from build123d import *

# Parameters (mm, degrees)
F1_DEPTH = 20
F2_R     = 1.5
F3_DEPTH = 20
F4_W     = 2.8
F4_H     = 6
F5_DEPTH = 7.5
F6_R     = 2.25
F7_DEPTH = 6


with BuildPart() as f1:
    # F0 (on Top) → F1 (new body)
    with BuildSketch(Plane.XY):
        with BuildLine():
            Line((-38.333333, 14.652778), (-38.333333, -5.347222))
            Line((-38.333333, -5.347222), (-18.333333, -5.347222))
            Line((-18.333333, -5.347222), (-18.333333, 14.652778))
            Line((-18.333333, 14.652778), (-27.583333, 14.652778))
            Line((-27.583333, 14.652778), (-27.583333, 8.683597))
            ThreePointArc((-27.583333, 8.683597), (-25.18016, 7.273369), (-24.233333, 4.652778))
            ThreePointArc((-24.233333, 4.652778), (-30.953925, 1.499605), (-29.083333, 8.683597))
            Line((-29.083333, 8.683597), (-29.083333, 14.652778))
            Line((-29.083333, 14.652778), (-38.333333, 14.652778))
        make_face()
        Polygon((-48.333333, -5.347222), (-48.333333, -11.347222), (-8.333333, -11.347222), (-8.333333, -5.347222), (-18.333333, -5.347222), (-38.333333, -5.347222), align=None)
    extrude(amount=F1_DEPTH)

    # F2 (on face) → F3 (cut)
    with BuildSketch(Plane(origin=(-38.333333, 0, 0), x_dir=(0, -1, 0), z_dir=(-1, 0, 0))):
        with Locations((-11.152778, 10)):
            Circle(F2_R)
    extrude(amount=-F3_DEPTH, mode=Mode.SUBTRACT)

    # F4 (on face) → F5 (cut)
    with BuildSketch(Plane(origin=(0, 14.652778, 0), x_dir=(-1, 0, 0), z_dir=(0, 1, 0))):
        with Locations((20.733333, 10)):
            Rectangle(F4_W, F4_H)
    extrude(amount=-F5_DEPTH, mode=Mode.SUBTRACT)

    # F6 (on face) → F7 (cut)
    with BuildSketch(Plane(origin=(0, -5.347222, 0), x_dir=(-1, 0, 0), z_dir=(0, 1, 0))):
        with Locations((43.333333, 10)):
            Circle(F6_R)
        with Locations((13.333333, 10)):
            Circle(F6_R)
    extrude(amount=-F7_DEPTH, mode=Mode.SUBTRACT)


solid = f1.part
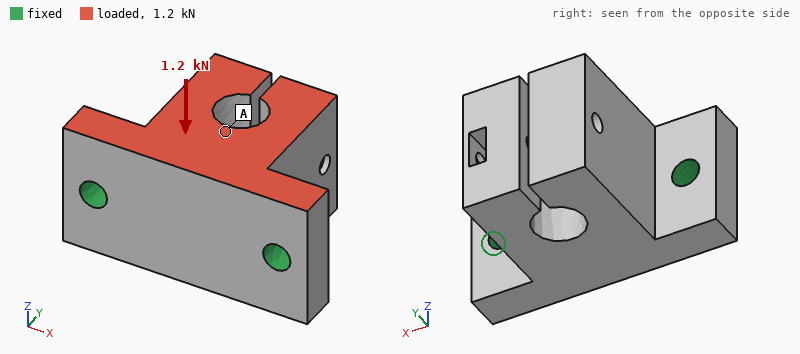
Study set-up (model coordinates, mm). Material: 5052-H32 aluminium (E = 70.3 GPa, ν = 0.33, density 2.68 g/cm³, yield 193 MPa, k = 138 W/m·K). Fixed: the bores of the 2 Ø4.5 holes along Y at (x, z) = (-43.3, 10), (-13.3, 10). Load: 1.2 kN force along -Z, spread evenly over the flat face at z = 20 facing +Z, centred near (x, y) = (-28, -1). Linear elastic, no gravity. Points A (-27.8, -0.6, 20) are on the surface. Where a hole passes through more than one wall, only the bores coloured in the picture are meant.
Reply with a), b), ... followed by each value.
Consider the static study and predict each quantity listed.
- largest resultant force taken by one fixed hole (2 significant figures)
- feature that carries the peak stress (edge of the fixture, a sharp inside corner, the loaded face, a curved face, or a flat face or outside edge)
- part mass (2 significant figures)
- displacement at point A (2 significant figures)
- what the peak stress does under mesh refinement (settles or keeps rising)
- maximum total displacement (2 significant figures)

a) 600 N
b) edge of the fixture
c) 30 g
d) 13 µm
e) keeps rising
f) 26 µm
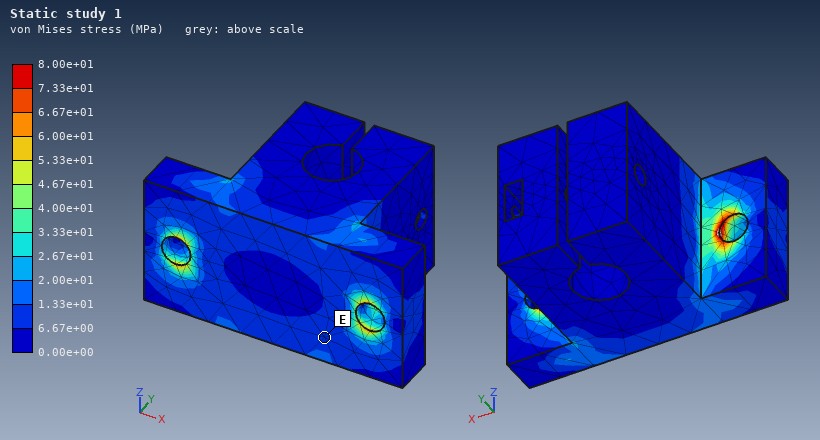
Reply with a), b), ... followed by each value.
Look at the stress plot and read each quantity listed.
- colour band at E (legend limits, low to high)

a) 6.67e+00 to 1.33e+01 MPa
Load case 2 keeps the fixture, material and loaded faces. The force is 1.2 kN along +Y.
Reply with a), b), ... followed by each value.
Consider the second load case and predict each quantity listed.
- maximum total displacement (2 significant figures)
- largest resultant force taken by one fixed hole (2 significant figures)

a) 29 µm
b) 630 N
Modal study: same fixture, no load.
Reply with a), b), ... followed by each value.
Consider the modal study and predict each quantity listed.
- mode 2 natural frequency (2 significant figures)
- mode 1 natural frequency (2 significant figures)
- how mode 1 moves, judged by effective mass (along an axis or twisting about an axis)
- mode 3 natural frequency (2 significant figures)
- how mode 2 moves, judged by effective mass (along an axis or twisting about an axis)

a) 13 kHz
b) 7400 Hz
c) along Z
d) 15 kHz
e) along X
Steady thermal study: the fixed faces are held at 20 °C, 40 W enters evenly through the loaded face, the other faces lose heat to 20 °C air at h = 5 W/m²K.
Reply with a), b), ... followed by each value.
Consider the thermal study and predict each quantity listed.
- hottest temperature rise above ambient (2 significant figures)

a) 19 K
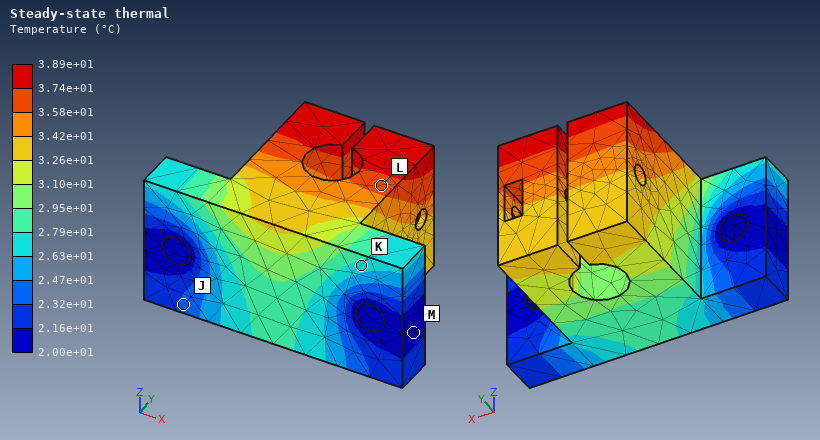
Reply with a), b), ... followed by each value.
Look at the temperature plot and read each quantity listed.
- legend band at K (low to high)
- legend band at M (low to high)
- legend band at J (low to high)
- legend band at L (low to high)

a) 2.63e+01 to 2.79e+01 °C
b) 2.00e+01 to 2.16e+01 °C
c) 2.32e+01 to 2.47e+01 °C
d) 3.58e+01 to 3.74e+01 °C
